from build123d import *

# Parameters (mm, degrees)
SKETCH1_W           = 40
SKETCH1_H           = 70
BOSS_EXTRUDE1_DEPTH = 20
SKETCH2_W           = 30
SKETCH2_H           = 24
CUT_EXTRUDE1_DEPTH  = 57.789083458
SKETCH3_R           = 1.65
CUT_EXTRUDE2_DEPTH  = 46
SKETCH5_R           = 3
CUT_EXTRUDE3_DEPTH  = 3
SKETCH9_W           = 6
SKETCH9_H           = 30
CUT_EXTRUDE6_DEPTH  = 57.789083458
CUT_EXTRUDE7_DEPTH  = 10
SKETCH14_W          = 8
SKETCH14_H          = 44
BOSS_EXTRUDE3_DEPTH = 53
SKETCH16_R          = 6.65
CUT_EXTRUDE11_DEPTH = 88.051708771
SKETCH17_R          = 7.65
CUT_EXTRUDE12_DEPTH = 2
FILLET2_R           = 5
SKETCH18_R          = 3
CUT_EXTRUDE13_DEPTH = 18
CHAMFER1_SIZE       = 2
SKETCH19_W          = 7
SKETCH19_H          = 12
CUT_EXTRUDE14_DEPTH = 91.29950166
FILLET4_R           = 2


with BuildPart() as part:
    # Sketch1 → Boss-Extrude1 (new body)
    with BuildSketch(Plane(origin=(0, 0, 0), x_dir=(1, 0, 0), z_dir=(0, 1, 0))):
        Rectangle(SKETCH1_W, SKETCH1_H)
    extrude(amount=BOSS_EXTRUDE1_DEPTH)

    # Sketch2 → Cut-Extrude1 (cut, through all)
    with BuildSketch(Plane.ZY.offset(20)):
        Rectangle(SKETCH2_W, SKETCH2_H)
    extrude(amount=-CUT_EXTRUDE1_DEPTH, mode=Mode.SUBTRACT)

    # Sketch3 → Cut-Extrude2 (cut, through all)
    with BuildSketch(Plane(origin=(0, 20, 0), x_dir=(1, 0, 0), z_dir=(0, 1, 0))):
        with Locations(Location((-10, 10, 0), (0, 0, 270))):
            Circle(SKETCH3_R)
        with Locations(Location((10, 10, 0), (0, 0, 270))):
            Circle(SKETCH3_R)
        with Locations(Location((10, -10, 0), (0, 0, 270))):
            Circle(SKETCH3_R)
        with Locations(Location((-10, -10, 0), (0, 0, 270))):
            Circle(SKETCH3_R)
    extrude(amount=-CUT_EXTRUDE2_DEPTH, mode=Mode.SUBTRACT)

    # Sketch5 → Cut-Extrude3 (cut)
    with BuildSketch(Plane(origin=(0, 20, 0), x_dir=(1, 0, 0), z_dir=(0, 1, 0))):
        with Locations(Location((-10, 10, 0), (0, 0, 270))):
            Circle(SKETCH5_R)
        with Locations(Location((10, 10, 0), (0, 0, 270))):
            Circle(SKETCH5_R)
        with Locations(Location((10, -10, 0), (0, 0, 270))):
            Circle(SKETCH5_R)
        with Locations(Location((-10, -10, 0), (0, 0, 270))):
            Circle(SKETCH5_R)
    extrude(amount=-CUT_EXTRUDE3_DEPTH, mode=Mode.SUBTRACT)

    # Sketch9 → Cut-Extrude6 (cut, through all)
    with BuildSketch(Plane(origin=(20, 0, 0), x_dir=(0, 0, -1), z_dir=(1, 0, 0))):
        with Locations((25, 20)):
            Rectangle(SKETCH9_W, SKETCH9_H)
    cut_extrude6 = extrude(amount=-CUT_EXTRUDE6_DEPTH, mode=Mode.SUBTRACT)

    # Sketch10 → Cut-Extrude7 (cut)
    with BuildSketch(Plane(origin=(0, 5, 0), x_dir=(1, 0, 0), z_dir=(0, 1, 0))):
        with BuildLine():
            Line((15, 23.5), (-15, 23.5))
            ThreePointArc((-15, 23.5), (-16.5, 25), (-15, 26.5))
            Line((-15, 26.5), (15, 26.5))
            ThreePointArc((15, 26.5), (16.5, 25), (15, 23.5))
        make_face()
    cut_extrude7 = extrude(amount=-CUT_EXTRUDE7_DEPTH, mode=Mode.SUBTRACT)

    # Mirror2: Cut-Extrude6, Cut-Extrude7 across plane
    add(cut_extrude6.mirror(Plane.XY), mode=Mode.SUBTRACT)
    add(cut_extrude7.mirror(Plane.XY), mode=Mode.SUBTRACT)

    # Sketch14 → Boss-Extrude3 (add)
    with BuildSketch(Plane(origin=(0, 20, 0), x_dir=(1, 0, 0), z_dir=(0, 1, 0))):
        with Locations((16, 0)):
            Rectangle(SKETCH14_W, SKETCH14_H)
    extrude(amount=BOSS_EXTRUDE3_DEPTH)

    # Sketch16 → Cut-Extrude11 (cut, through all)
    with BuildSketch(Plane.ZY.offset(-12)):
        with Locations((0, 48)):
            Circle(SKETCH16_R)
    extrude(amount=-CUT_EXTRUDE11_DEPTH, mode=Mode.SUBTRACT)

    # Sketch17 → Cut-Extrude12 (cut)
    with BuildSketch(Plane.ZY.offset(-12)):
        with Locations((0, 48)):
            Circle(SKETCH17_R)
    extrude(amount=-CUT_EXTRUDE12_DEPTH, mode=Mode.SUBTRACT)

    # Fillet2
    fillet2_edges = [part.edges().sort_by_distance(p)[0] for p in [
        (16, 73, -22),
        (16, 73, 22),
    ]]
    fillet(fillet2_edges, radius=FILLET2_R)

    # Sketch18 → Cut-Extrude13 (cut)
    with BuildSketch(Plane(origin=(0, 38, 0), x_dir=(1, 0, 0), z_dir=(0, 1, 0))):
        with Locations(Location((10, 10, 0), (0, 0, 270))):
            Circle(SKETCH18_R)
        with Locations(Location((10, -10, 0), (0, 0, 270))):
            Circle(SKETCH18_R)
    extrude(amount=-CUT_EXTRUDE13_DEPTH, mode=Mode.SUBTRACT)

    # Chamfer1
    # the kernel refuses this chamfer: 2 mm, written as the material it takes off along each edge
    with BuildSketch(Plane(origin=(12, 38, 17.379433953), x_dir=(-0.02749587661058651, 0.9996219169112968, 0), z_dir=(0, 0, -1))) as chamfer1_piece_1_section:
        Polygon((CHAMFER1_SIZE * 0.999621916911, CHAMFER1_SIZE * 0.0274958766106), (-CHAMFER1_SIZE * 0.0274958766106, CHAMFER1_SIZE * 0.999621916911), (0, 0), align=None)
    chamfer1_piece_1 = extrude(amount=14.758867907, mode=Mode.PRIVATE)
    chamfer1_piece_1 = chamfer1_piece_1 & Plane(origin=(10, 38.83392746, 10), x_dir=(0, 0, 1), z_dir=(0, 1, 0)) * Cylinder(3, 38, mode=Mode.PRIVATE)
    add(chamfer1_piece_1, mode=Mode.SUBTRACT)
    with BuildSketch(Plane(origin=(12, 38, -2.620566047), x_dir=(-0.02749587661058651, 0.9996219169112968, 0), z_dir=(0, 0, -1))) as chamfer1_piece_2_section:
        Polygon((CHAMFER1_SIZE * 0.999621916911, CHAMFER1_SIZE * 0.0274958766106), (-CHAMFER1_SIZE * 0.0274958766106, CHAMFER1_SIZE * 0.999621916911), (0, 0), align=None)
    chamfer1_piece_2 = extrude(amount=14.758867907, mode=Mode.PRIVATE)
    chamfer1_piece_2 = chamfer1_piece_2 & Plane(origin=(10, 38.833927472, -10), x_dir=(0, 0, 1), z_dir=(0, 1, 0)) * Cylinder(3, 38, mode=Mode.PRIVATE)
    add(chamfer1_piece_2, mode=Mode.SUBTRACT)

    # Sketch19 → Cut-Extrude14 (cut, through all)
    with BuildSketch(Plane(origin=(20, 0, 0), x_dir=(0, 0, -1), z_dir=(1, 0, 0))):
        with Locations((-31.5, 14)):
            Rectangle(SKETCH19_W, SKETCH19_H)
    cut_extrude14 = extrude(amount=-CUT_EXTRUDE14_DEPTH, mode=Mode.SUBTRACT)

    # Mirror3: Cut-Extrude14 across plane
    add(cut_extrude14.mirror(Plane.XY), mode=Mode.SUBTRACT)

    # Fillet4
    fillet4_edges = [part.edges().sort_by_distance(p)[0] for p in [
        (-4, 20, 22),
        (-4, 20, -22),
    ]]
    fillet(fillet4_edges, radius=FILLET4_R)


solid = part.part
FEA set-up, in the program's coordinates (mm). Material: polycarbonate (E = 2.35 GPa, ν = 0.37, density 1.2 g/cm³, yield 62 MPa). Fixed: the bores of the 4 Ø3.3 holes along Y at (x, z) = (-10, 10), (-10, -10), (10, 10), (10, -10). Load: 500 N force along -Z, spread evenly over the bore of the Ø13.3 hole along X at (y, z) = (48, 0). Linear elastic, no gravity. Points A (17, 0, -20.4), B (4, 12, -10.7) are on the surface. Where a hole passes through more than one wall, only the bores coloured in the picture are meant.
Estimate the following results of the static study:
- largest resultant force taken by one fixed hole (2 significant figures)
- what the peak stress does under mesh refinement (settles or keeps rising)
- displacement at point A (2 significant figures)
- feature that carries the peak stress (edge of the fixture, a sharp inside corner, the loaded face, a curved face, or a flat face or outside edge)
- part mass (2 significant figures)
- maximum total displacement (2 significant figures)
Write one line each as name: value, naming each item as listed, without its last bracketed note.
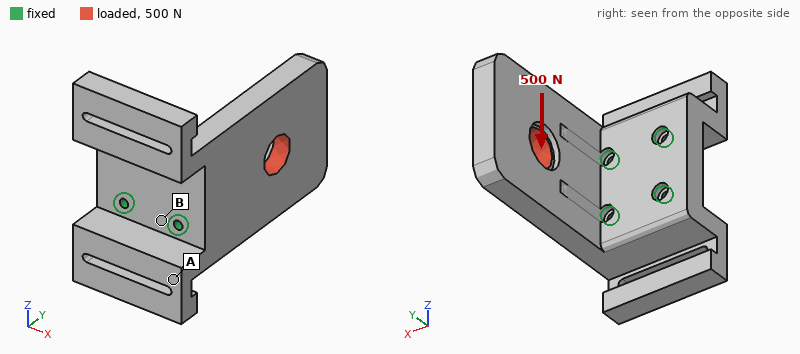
largest resultant force taken by one fixed hole: 730 N
what the peak stress does under mesh refinement: keeps rising
displacement at point A: 0.19 mm
feature that carries the peak stress: edge of the fixture
part mass: 52 g
maximum total displacement: 0.60 mm
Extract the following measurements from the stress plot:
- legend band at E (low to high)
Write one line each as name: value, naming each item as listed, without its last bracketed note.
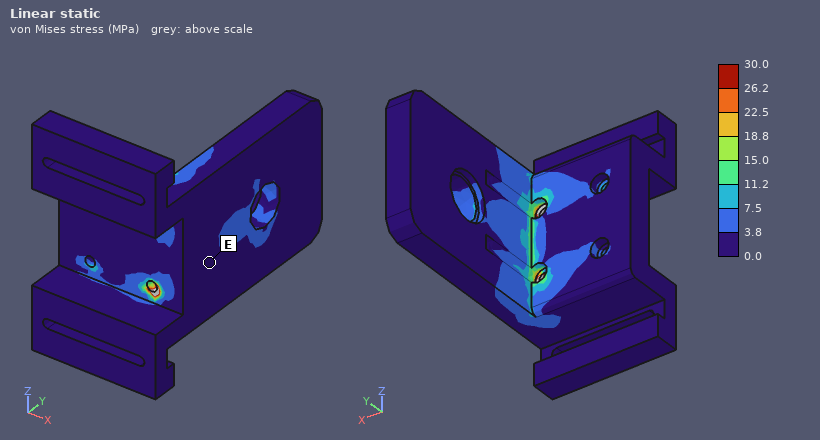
legend band at E: 0.0 to 3.8 MPa
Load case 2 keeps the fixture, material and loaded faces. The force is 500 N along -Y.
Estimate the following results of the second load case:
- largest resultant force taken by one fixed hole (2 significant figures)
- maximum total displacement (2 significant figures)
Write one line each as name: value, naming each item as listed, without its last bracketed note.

largest resultant force taken by one fixed hole: 310 N
maximum total displacement: 0.41 mm
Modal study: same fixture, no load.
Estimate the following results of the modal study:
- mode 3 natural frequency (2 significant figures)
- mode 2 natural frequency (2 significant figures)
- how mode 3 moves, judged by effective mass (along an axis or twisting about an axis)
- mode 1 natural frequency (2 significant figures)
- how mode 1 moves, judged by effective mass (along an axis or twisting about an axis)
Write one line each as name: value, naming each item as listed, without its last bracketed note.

mode 3 natural frequency: 1300 Hz
mode 2 natural frequency: 1100 Hz
how mode 3 moves, judged by effective mass: along Y
mode 1 natural frequency: 480 Hz
how mode 1 moves, judged by effective mass: along X
